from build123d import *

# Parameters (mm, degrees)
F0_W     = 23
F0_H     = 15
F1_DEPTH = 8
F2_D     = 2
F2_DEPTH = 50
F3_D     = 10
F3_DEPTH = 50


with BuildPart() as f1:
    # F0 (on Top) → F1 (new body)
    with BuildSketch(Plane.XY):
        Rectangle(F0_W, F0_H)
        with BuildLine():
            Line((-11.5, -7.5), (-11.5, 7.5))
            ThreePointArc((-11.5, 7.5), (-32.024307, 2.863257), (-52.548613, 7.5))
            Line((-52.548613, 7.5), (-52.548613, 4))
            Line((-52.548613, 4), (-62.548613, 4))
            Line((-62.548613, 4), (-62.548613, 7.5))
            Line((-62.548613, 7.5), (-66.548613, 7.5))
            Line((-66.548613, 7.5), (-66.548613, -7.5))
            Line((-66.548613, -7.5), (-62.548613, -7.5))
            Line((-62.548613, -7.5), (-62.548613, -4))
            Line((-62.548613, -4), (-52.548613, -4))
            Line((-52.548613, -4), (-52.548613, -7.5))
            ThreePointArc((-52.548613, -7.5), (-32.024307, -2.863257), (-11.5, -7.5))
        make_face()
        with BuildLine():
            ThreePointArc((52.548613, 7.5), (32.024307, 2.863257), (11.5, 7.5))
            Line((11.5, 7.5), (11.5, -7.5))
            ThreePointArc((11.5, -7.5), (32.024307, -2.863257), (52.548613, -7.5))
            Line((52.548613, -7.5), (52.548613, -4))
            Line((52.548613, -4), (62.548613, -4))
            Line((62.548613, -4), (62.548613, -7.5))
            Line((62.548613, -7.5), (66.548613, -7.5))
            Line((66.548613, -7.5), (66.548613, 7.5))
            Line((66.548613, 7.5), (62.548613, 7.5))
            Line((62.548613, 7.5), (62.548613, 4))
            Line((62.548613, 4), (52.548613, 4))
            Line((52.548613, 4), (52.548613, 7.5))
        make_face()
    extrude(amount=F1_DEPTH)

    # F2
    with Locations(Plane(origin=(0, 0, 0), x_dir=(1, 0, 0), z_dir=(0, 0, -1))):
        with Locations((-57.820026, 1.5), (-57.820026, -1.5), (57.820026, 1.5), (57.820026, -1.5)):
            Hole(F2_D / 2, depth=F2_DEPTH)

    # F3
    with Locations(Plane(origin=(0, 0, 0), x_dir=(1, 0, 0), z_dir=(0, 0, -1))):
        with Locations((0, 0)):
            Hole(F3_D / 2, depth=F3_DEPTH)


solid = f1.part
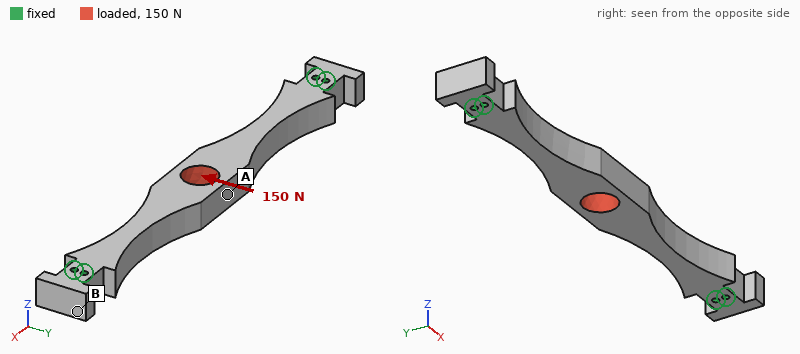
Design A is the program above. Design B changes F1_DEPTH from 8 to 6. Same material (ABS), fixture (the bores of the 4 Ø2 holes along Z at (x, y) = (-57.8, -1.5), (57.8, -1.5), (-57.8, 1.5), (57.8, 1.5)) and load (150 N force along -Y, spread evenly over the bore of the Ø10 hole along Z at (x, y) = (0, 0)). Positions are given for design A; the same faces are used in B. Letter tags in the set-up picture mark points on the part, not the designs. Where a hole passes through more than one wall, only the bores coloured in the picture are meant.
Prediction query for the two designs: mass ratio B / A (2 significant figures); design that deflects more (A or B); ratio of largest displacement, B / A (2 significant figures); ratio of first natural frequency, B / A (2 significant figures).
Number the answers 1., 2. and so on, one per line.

1. 0.75
2. B
3. 1.3
4. 0.77
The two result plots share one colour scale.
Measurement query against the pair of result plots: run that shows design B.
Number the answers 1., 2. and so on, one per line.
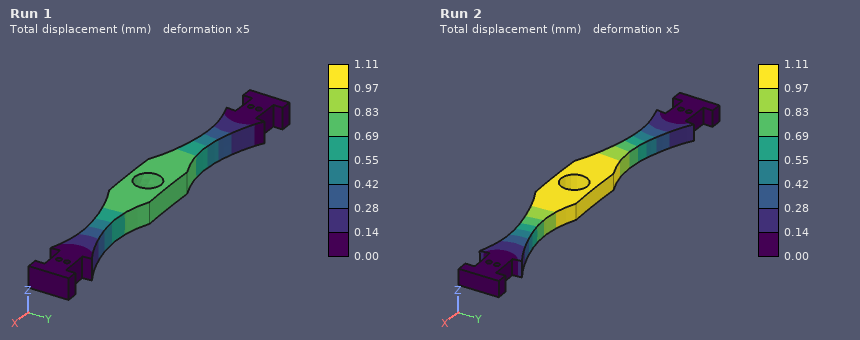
1. Run 2
